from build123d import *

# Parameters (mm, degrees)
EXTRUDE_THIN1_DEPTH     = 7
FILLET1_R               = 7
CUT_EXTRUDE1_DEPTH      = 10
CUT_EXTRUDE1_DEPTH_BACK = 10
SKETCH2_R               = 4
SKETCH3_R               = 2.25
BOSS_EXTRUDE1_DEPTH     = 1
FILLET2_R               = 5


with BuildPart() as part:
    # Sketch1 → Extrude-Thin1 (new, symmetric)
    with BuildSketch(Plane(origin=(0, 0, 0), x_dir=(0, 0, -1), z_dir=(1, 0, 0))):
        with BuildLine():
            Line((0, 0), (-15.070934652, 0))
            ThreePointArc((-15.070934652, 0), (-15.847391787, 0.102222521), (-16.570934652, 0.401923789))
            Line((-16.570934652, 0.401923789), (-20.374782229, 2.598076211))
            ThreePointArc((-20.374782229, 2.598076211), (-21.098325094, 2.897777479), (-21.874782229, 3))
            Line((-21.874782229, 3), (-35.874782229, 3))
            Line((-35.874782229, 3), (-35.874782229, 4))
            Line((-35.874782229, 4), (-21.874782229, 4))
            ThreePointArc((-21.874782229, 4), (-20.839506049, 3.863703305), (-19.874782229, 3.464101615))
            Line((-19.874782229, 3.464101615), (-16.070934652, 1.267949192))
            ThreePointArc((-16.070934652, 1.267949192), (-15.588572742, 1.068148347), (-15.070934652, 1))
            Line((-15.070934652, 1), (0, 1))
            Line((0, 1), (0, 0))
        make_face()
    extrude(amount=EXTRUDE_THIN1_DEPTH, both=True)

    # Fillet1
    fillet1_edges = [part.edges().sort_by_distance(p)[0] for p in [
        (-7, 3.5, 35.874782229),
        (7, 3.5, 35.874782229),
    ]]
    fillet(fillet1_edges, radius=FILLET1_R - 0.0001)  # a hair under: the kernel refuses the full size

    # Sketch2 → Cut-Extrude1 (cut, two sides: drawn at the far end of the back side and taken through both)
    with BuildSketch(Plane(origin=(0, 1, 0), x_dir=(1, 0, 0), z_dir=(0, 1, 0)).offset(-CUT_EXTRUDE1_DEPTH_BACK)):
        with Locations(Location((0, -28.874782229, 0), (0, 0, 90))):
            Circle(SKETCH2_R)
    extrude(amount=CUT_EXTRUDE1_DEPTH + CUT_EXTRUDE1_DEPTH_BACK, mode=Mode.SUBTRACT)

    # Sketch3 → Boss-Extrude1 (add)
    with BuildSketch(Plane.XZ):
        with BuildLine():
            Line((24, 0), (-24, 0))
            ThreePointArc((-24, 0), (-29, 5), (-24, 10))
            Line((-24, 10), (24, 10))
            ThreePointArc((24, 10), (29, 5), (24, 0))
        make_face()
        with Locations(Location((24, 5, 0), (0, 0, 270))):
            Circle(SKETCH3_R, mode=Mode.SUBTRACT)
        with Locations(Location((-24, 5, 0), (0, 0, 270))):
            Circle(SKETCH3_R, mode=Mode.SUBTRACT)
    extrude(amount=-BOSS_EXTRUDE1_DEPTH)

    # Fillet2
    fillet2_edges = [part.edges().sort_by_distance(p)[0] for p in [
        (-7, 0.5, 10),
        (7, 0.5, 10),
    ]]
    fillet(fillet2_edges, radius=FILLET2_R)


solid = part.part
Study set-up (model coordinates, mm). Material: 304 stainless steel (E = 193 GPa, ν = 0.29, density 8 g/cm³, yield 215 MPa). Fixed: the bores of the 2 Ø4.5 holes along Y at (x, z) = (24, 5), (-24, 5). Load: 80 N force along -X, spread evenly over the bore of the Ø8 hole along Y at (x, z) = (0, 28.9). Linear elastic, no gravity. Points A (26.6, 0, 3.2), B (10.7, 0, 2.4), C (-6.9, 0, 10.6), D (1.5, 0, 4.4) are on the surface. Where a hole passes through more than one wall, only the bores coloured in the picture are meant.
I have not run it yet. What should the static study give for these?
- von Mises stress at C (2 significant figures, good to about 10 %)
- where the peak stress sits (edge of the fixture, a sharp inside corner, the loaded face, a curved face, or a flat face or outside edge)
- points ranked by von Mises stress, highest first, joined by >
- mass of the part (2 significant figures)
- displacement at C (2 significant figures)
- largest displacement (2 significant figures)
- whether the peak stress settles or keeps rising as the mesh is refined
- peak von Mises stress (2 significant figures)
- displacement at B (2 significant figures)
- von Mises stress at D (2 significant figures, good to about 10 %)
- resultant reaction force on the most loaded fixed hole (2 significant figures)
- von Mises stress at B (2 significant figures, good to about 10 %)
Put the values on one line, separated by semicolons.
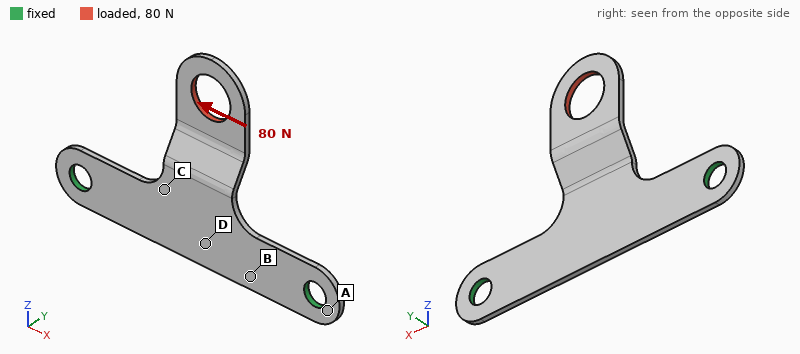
48 MPa; a curved face; C > D > B > A; 6.7 g; 16 µm; 42 µm; settles; 190 MPa; 6.4 µm; 36 MPa; 66 N; 25 MPa
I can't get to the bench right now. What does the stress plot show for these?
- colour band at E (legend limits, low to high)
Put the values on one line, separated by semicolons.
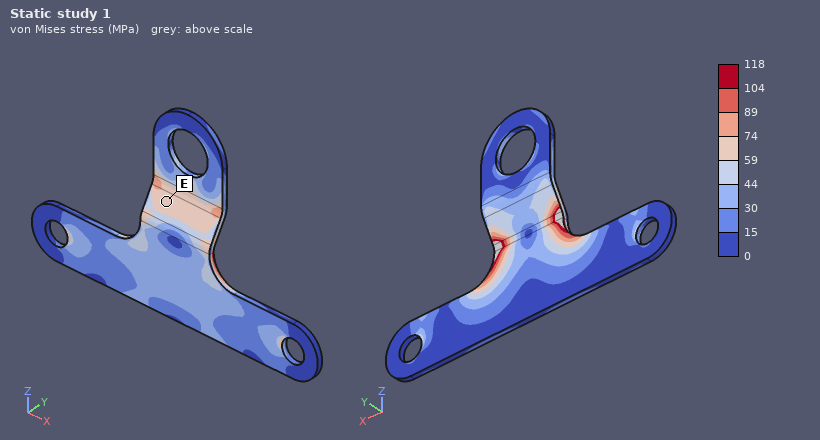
59 to 74 MPa
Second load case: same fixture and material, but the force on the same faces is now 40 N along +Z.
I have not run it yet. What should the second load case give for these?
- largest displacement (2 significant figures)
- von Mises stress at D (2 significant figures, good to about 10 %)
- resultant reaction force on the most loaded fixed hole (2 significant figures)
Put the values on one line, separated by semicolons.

0.23 mm; 12 MPa; 22 N
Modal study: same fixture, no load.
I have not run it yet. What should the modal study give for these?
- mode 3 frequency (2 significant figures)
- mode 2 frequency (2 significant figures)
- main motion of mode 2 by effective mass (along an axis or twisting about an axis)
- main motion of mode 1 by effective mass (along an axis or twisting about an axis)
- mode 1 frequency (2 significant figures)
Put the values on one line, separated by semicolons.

4000 Hz; 2400 Hz; along Y; along Y; 800 Hz
